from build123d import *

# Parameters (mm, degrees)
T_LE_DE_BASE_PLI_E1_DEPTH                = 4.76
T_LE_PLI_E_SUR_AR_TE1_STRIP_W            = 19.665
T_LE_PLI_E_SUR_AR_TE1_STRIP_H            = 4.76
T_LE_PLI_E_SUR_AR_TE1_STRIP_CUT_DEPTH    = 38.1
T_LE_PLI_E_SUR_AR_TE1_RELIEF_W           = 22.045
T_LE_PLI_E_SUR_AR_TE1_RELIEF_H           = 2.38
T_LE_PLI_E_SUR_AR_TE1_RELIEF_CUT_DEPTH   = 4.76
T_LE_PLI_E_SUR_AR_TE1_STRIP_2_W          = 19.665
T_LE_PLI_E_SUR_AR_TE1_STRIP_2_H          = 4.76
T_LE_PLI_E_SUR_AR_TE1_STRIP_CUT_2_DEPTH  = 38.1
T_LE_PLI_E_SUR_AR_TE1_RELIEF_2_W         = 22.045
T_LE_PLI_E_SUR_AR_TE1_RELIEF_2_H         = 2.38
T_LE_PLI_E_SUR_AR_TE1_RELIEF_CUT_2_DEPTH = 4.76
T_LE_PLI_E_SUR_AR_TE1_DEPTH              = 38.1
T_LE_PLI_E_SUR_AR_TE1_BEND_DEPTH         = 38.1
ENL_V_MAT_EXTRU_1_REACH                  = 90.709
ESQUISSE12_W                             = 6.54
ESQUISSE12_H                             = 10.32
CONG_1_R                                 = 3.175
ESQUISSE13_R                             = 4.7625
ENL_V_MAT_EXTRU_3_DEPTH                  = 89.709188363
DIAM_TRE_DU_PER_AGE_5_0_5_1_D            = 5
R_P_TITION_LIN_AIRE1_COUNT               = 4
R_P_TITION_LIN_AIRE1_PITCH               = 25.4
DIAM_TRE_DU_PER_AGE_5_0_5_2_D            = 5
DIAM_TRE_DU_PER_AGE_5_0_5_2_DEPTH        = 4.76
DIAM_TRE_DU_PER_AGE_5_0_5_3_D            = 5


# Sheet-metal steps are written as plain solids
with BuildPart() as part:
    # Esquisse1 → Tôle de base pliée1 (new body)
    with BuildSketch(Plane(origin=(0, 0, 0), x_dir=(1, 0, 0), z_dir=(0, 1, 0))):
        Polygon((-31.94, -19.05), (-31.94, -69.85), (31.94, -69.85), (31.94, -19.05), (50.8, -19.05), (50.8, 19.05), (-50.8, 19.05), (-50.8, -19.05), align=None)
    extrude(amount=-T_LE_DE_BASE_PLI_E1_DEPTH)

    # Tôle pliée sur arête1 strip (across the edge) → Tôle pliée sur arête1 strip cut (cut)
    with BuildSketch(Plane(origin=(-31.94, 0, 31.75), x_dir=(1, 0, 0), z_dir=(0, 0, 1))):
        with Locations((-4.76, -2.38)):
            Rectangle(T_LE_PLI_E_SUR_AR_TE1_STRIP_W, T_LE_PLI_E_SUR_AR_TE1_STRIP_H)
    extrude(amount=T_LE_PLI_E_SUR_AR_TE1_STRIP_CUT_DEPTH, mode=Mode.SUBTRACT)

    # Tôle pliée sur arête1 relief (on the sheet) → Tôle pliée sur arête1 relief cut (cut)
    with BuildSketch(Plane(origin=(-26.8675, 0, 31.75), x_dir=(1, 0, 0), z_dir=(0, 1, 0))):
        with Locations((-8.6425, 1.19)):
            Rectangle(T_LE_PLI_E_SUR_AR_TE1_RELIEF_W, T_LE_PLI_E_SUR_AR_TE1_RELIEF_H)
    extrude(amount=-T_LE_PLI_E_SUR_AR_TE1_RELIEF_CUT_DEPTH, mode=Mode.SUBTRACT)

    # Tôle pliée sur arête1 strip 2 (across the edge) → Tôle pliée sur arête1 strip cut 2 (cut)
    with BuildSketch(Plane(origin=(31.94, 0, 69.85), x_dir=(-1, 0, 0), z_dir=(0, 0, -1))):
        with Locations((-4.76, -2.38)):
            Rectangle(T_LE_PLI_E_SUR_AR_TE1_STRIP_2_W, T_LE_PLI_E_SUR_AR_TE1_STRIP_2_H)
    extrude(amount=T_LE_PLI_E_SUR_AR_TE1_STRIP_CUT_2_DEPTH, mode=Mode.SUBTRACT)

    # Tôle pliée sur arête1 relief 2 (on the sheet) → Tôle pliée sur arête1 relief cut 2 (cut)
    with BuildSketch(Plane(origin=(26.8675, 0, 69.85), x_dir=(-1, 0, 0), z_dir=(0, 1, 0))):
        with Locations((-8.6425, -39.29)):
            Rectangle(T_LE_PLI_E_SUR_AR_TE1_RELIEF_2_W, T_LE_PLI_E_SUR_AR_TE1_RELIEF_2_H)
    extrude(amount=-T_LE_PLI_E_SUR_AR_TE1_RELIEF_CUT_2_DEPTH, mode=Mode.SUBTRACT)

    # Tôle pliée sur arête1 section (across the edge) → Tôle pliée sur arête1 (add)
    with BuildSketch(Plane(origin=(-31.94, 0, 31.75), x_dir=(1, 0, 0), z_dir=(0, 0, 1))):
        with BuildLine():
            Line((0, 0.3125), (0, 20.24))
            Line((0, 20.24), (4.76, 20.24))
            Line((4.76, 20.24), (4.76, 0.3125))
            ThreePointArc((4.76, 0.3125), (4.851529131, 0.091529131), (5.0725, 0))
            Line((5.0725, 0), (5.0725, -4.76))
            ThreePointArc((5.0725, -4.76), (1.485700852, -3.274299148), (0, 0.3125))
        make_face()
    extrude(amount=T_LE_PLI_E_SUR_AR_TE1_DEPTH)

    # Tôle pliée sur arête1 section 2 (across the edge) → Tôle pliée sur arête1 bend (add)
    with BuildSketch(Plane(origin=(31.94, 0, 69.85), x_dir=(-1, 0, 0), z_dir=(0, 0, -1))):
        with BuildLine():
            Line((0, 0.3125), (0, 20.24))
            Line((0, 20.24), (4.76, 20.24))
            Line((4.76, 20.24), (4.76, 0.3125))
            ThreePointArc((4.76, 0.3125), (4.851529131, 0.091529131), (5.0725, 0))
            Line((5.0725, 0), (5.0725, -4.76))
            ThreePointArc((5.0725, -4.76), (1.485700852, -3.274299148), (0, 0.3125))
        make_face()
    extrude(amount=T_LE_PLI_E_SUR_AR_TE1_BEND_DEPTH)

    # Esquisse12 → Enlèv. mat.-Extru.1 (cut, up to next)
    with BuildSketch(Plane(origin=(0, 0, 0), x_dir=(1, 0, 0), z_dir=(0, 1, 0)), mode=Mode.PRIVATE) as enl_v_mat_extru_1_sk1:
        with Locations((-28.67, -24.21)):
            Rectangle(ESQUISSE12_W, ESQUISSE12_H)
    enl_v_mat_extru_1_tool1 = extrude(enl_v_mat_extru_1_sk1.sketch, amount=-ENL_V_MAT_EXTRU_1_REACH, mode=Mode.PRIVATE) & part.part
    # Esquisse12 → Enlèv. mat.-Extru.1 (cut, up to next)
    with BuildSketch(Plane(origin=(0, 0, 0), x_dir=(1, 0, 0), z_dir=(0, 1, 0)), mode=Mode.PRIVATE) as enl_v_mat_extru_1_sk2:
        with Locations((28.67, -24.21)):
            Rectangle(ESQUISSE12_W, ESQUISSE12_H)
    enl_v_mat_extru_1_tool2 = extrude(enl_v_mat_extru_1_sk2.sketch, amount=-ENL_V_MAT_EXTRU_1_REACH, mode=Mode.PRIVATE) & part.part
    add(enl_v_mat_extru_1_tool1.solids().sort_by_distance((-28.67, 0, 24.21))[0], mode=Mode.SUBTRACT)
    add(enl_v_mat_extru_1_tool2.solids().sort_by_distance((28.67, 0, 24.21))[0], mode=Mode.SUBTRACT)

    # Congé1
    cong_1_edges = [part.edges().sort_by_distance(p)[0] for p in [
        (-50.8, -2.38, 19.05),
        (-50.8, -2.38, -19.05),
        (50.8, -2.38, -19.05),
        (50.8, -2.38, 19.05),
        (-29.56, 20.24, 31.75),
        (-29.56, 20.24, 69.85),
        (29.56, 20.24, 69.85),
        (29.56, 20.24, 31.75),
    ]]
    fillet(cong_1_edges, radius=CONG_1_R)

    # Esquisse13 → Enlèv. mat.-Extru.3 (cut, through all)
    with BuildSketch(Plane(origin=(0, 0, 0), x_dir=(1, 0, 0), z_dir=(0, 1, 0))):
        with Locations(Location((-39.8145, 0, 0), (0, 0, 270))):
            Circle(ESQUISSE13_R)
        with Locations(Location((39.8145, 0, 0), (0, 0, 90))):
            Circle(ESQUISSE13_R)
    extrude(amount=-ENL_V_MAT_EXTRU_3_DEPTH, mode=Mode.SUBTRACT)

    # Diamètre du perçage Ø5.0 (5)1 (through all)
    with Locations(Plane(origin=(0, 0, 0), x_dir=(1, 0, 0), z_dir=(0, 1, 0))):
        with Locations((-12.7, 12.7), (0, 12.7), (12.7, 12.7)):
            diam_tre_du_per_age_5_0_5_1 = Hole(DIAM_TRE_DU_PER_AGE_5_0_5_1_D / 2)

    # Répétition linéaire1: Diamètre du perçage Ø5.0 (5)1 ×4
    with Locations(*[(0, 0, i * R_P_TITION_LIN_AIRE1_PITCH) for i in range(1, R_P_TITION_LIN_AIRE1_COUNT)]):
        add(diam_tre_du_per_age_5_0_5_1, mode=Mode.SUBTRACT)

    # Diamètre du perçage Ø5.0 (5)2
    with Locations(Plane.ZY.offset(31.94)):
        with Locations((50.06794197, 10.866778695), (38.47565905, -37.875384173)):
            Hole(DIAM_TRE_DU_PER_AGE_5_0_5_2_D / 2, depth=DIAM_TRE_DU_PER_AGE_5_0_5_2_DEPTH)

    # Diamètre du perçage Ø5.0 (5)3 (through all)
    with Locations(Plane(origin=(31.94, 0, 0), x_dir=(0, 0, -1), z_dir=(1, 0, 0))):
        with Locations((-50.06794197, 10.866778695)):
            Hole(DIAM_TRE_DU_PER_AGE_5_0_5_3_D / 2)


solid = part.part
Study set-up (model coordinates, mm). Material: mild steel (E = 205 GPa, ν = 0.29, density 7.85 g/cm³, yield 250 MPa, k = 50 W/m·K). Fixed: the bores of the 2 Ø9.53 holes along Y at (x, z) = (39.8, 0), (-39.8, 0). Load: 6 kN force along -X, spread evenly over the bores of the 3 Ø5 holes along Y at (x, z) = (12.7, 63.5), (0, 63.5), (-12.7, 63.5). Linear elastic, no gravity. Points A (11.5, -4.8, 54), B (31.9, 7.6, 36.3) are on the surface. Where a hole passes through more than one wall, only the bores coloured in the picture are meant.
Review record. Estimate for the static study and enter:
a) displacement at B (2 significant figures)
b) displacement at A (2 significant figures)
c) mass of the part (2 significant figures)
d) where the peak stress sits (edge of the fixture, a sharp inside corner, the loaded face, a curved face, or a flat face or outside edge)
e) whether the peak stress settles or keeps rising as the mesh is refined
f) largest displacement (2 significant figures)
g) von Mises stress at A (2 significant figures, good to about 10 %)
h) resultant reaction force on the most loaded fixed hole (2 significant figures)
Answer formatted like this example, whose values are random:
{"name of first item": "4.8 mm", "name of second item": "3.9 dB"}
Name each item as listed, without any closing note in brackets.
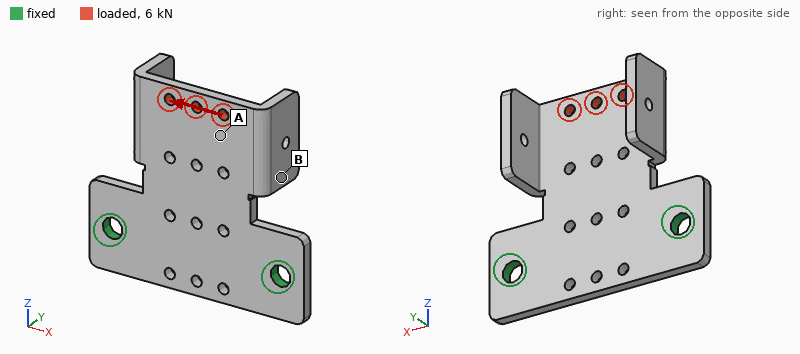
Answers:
{"displacement at B": "42 µm", "displacement at A": "49 µm", "mass of the part": "300 g", "where the peak stress sits": "a sharp inside corner", "whether the peak stress settles or keeps rising as the mesh is refined": "keeps rising", "largest displacement": "76 µm", "von Mises stress at A": "52 MPa", "resultant reaction force on the most loaded fixed hole": "5.8 kN"}
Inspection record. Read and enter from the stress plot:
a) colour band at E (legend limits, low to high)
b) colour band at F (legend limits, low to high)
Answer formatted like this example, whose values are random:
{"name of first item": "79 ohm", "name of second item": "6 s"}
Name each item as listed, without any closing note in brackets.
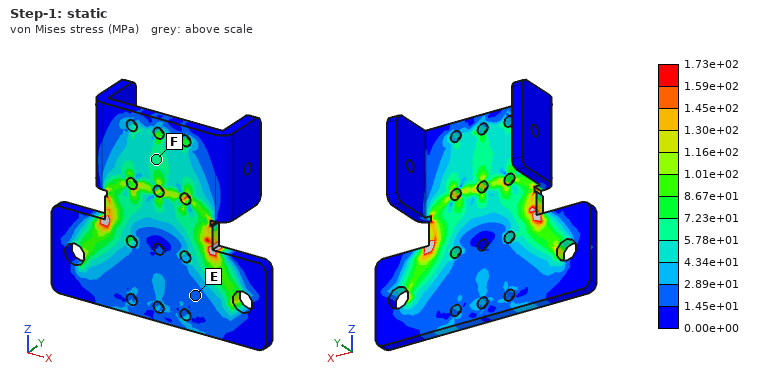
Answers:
{"colour band at E": "1.45e+01 to 2.89e+01 MPa", "colour band at F": "5.78e+01 to 7.23e+01 MPa"}
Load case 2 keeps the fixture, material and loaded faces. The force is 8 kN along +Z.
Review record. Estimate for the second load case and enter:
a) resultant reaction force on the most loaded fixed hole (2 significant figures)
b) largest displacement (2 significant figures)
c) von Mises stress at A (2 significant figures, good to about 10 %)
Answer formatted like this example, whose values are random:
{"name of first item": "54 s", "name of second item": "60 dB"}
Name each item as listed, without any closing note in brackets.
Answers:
{"resultant reaction force on the most loaded fixed hole": "4.2 kN", "largest displacement": "21 µm", "von Mises stress at A": "40 MPa"}
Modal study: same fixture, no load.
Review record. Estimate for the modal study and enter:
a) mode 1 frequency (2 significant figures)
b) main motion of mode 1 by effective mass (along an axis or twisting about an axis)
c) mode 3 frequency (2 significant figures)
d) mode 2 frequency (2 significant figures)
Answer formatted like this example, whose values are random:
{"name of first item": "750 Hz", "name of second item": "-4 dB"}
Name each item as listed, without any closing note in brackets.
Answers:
{"mode 1 frequency": "550 Hz", "main motion of mode 1 by effective mass": "along Y", "mode 3 frequency": "2900 Hz", "mode 2 frequency": "1200 Hz"}
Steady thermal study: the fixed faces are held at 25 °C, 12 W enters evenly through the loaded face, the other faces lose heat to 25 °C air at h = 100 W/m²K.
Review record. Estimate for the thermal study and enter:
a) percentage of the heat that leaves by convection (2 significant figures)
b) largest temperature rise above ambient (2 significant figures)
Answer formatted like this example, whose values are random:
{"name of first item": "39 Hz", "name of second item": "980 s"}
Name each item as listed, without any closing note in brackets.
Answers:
{"percentage of the heat that leaves by convection": "90 %", "largest temperature rise above ambient": "26 K"}
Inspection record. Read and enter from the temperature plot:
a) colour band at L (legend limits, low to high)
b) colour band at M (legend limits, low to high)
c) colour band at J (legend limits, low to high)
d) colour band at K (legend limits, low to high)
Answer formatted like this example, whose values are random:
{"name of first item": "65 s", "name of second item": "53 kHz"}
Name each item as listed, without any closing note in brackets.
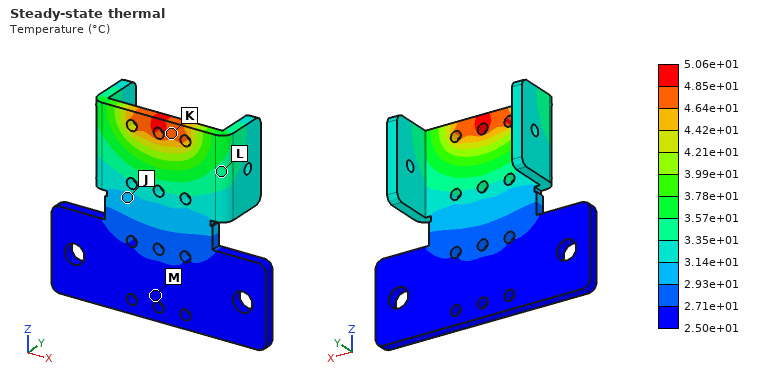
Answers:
{"colour band at L": "3.35e+01 to 3.57e+01 °C", "colour band at M": "2.50e+01 to 2.71e+01 °C", "colour band at J": "2.93e+01 to 3.14e+01 °C", "colour band at K": "4.64e+01 to 4.85e+01 °C"}
